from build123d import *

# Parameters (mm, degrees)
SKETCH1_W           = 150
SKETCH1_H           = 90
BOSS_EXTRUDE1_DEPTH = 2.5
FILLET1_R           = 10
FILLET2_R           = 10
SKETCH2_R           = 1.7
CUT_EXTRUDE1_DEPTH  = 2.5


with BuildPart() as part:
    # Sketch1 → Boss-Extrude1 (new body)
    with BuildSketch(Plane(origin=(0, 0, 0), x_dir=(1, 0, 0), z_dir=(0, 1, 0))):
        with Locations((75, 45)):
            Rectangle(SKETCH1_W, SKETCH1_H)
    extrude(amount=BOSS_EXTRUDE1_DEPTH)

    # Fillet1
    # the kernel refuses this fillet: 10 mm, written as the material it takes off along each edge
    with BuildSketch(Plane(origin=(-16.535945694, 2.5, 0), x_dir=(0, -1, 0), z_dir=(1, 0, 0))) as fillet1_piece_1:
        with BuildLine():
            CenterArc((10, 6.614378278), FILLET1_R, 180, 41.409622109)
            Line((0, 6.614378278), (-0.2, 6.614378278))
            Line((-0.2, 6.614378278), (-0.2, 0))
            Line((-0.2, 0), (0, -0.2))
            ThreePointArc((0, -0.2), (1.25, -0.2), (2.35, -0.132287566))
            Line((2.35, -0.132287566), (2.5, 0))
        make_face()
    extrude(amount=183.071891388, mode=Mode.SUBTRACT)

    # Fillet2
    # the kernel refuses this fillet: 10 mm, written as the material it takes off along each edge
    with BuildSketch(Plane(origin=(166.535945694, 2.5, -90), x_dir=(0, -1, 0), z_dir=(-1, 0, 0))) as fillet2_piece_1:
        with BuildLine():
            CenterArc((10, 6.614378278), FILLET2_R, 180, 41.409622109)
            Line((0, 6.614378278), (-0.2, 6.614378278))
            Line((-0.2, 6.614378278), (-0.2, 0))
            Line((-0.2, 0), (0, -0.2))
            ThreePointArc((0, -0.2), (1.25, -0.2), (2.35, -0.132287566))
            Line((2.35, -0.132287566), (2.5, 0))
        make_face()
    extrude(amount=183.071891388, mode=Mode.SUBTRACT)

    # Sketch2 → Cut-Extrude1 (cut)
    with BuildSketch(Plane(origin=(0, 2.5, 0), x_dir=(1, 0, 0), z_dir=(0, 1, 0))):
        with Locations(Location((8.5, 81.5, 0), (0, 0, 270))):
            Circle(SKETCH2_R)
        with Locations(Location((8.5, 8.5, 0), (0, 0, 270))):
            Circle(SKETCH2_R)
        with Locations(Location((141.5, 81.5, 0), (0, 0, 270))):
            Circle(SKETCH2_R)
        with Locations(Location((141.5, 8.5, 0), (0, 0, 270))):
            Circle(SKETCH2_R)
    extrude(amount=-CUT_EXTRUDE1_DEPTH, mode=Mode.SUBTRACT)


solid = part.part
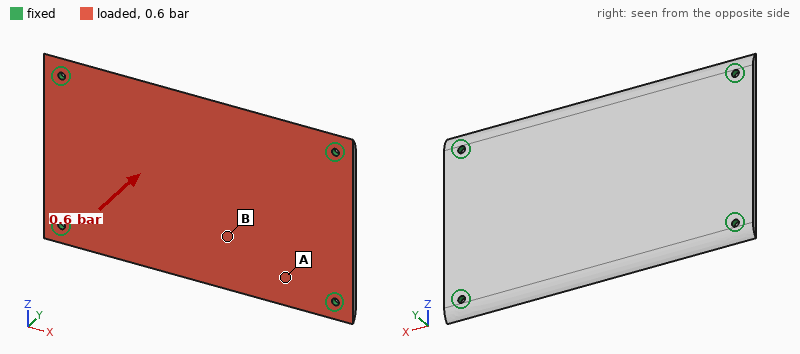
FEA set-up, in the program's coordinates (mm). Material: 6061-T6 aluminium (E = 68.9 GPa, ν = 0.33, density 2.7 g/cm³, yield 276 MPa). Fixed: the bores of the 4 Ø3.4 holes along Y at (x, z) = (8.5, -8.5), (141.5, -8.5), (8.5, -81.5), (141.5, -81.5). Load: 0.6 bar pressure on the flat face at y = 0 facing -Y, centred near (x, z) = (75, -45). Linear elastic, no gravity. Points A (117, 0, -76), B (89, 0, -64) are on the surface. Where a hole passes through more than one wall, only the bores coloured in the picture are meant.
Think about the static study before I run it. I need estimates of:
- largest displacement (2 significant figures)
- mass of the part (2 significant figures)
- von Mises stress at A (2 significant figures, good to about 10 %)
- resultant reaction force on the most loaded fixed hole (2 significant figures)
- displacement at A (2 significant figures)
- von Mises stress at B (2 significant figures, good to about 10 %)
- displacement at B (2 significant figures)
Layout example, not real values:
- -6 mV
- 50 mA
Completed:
- 0.85 mm
- 87 g
- 17 MPa
- 200 N
- 0.34 mm
- 44 MPa
- 0.76 mm
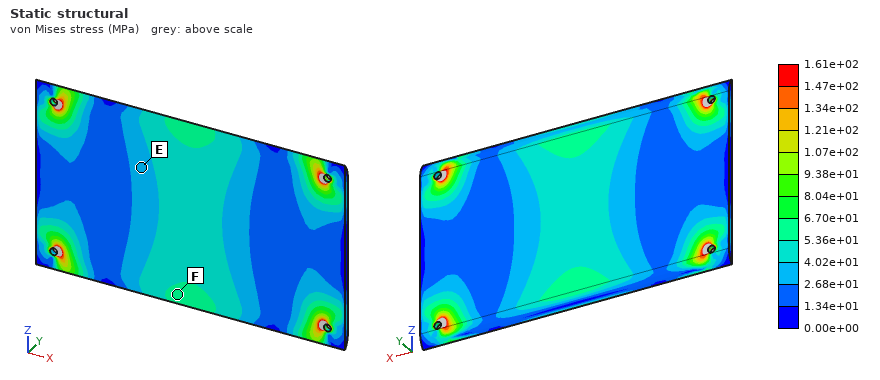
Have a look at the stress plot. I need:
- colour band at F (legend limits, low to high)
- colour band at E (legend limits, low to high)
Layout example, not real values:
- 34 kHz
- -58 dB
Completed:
- 5.36e+01 to 6.70e+01 MPa
- 2.68e+01 to 4.02e+01 MPa
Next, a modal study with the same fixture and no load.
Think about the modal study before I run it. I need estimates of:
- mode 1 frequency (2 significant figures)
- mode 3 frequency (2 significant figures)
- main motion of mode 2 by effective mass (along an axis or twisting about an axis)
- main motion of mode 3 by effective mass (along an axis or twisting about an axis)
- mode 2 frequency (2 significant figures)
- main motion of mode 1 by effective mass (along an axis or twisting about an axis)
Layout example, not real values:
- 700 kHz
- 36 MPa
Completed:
- 610 Hz
- 1600 Hz
- twisting about X
- twisting about Z
- 1000 Hz
- along Y
